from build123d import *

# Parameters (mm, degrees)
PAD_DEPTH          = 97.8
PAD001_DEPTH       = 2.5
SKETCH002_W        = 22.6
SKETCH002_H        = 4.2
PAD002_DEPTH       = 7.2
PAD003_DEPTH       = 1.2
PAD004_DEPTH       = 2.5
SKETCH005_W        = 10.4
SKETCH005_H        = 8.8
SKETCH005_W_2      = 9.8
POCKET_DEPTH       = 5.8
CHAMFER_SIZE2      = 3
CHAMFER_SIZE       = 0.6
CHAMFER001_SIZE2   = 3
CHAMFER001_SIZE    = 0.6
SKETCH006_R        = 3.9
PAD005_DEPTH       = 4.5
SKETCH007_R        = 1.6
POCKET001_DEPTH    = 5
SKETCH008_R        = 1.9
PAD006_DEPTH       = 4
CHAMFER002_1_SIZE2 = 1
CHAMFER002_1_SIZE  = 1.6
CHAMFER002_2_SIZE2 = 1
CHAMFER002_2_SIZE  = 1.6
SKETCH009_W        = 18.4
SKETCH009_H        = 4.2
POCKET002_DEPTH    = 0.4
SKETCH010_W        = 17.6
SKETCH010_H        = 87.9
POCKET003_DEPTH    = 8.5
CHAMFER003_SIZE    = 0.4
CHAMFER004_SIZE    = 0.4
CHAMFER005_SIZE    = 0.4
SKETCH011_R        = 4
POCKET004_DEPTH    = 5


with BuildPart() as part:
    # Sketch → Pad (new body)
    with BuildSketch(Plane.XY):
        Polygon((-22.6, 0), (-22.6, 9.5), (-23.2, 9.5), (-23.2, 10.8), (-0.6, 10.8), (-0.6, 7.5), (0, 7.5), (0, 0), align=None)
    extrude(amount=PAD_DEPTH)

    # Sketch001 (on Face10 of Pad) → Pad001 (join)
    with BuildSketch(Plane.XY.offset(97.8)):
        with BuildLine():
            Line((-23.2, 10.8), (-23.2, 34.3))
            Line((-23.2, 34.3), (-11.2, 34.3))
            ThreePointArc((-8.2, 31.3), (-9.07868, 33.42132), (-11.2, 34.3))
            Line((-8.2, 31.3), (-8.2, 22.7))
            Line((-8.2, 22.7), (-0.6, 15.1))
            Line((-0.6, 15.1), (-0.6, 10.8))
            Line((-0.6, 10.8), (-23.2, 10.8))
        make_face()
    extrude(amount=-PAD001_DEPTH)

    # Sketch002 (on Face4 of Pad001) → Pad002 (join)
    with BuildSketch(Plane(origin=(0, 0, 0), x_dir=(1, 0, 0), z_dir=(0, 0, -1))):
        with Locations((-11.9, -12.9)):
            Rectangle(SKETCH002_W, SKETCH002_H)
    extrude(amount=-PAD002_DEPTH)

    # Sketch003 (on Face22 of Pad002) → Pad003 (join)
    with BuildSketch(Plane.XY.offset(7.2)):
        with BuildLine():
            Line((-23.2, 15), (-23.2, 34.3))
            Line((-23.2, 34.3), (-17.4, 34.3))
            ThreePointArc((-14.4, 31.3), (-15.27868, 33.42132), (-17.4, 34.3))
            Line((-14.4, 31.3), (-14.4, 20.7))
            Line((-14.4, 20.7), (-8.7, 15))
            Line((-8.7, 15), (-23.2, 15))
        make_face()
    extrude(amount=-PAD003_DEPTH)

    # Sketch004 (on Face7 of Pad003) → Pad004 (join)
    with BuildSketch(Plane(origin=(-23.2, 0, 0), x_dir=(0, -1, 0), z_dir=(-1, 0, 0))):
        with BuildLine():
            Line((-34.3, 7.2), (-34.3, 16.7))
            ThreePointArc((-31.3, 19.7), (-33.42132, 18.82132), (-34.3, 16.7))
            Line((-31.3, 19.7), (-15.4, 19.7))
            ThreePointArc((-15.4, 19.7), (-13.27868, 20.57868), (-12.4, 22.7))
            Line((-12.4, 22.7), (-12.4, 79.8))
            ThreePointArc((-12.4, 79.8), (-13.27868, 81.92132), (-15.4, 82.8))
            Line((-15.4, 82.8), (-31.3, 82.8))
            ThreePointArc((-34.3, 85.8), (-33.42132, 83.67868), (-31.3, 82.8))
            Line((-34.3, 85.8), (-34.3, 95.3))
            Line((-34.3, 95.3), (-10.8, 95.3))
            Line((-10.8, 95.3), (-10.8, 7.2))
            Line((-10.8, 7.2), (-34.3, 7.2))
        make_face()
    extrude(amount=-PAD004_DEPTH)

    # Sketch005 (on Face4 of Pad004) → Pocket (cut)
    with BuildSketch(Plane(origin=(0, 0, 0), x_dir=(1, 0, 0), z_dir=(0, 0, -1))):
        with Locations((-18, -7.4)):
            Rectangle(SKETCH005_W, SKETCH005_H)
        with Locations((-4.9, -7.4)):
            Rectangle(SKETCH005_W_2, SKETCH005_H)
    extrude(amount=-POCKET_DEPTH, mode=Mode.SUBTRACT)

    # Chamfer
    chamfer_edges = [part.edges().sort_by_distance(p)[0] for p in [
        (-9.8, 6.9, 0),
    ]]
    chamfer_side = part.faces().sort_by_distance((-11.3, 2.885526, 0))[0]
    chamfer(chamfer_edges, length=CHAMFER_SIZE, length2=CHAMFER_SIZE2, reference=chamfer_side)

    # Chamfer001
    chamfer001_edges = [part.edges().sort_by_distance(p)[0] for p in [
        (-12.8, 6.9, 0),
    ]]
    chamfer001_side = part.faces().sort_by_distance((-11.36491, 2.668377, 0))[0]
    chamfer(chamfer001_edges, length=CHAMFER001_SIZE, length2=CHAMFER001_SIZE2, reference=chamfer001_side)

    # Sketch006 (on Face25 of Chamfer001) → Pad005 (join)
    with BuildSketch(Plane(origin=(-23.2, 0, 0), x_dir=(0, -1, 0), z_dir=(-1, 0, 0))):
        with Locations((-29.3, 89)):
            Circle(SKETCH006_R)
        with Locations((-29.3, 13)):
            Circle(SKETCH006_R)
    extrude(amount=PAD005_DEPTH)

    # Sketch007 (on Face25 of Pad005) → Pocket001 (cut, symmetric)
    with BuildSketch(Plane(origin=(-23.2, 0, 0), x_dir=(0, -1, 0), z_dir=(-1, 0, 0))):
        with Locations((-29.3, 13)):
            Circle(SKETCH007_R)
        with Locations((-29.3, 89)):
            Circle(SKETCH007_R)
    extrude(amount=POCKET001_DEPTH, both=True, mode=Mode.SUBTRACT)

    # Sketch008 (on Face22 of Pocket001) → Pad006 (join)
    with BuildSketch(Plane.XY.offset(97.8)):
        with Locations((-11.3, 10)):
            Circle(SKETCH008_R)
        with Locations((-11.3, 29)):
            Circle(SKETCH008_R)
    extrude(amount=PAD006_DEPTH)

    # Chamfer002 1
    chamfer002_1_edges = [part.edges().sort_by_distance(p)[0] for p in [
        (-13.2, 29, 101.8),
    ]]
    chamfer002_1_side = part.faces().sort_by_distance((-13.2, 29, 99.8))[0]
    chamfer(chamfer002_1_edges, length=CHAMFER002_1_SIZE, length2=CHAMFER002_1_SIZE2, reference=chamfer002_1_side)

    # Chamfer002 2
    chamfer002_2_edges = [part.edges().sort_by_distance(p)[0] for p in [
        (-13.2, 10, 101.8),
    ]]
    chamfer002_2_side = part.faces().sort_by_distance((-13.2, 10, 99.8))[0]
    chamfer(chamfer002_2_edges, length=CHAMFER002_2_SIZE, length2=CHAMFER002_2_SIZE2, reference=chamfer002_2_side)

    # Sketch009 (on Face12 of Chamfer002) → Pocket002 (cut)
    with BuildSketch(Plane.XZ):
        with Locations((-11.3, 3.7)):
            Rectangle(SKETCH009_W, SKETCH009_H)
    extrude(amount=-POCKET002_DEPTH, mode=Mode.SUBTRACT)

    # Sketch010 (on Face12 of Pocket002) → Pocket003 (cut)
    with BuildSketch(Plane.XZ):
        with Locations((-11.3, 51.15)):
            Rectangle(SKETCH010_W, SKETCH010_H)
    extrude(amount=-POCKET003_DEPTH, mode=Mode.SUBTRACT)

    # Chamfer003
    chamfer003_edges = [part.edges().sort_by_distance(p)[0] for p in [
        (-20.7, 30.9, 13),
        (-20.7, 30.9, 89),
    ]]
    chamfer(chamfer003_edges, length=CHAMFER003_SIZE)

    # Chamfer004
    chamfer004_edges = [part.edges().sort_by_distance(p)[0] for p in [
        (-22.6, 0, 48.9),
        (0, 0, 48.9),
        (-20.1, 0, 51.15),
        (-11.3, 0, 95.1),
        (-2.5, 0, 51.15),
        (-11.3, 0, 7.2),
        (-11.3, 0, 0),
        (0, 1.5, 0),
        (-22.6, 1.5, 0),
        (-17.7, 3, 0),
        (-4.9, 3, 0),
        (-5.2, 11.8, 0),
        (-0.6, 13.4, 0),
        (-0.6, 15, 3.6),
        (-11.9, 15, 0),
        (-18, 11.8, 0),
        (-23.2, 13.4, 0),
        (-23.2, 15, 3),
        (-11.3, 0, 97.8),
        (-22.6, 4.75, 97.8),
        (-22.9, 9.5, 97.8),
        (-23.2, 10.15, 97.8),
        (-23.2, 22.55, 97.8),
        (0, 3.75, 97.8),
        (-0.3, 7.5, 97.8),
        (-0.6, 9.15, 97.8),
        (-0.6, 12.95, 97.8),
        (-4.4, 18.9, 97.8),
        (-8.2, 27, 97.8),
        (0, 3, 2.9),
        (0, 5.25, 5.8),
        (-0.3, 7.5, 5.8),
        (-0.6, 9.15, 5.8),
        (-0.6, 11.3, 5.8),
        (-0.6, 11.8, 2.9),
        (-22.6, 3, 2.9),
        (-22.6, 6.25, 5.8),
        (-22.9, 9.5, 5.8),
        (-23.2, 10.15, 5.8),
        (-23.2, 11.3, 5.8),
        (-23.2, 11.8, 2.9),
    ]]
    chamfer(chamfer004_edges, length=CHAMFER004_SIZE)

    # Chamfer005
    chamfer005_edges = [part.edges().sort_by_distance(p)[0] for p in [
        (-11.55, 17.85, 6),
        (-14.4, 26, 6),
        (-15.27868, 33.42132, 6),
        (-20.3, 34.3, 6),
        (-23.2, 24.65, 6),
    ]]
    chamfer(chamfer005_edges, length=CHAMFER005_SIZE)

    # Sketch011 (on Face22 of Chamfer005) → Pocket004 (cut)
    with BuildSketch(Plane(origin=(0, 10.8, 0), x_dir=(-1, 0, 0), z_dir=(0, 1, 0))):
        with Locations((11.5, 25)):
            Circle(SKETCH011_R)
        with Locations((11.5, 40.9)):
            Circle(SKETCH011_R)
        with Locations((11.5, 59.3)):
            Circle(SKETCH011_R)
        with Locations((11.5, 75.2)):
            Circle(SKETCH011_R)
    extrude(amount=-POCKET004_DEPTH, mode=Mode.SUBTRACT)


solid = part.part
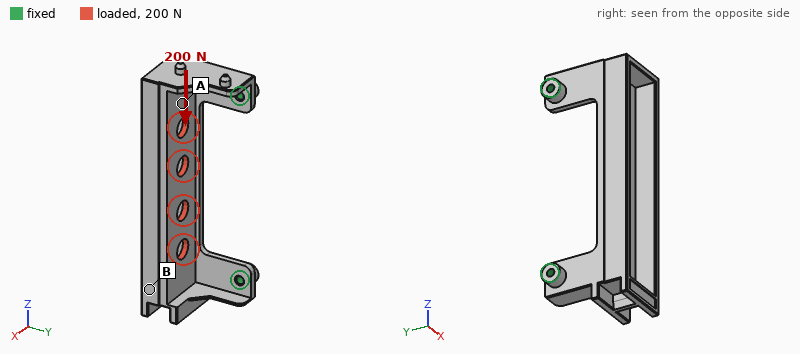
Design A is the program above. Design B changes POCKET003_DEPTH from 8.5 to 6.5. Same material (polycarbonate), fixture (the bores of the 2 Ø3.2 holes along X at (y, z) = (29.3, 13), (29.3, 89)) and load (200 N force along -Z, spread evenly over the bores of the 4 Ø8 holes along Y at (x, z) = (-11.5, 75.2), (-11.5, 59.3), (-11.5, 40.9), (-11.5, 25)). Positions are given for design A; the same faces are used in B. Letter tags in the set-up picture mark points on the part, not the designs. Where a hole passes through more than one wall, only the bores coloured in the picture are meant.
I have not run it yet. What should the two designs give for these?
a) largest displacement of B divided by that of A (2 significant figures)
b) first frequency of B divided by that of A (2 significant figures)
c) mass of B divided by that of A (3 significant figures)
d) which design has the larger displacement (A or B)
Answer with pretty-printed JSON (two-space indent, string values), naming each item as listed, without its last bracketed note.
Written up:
{
  "largest displacement of B divided by that of A": "0.82",
  "first frequency of B divided by that of A": "0.91",
  "mass of B divided by that of A": "1.21",
  "which design has the larger displacement": "A"
}
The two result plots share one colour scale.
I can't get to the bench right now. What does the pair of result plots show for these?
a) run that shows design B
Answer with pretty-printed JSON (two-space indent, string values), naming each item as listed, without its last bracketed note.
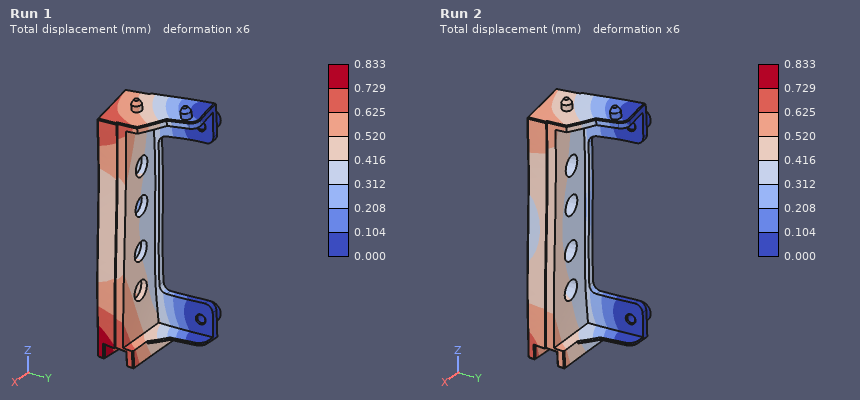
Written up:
{
  "run that shows design B": "Run 2"
}
